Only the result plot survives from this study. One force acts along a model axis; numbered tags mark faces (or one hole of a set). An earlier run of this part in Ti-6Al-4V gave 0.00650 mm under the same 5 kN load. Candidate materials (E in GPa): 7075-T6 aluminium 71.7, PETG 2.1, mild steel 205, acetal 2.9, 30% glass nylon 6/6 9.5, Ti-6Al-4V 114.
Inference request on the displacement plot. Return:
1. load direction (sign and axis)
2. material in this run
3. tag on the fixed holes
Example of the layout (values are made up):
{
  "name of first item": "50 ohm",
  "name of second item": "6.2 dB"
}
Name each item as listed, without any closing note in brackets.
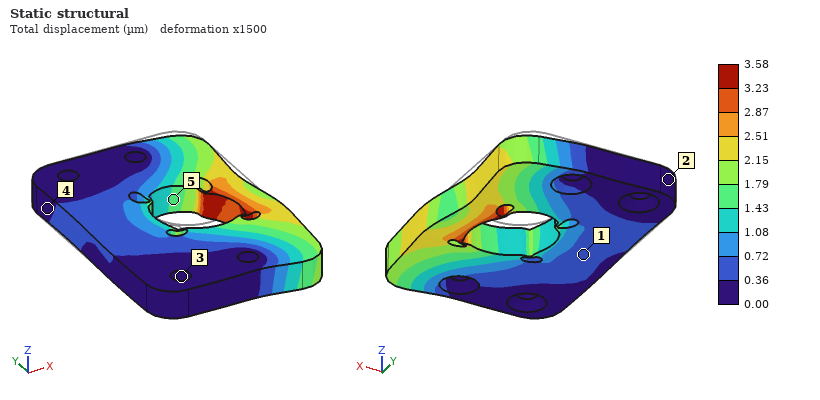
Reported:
{
  "load direction": "-Y",
  "material in this run": "mild steel",
  "tag on the fixed holes": "3"
}
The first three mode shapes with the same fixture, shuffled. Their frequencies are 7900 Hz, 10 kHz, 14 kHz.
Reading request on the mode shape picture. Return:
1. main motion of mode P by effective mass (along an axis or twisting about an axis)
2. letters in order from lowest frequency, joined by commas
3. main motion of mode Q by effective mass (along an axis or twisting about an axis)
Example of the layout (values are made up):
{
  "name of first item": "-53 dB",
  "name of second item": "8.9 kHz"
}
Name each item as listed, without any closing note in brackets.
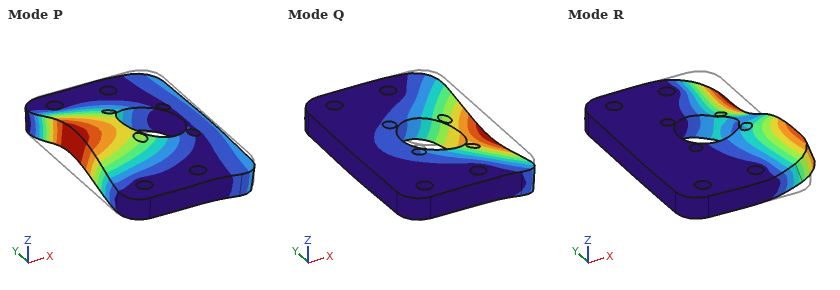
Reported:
{
  "main motion of mode P by effective mass": "along Z",
  "letters in order from lowest frequency, joined by commas": "Q, P, R",
  "main motion of mode Q by effective mass": "along Z"
}
